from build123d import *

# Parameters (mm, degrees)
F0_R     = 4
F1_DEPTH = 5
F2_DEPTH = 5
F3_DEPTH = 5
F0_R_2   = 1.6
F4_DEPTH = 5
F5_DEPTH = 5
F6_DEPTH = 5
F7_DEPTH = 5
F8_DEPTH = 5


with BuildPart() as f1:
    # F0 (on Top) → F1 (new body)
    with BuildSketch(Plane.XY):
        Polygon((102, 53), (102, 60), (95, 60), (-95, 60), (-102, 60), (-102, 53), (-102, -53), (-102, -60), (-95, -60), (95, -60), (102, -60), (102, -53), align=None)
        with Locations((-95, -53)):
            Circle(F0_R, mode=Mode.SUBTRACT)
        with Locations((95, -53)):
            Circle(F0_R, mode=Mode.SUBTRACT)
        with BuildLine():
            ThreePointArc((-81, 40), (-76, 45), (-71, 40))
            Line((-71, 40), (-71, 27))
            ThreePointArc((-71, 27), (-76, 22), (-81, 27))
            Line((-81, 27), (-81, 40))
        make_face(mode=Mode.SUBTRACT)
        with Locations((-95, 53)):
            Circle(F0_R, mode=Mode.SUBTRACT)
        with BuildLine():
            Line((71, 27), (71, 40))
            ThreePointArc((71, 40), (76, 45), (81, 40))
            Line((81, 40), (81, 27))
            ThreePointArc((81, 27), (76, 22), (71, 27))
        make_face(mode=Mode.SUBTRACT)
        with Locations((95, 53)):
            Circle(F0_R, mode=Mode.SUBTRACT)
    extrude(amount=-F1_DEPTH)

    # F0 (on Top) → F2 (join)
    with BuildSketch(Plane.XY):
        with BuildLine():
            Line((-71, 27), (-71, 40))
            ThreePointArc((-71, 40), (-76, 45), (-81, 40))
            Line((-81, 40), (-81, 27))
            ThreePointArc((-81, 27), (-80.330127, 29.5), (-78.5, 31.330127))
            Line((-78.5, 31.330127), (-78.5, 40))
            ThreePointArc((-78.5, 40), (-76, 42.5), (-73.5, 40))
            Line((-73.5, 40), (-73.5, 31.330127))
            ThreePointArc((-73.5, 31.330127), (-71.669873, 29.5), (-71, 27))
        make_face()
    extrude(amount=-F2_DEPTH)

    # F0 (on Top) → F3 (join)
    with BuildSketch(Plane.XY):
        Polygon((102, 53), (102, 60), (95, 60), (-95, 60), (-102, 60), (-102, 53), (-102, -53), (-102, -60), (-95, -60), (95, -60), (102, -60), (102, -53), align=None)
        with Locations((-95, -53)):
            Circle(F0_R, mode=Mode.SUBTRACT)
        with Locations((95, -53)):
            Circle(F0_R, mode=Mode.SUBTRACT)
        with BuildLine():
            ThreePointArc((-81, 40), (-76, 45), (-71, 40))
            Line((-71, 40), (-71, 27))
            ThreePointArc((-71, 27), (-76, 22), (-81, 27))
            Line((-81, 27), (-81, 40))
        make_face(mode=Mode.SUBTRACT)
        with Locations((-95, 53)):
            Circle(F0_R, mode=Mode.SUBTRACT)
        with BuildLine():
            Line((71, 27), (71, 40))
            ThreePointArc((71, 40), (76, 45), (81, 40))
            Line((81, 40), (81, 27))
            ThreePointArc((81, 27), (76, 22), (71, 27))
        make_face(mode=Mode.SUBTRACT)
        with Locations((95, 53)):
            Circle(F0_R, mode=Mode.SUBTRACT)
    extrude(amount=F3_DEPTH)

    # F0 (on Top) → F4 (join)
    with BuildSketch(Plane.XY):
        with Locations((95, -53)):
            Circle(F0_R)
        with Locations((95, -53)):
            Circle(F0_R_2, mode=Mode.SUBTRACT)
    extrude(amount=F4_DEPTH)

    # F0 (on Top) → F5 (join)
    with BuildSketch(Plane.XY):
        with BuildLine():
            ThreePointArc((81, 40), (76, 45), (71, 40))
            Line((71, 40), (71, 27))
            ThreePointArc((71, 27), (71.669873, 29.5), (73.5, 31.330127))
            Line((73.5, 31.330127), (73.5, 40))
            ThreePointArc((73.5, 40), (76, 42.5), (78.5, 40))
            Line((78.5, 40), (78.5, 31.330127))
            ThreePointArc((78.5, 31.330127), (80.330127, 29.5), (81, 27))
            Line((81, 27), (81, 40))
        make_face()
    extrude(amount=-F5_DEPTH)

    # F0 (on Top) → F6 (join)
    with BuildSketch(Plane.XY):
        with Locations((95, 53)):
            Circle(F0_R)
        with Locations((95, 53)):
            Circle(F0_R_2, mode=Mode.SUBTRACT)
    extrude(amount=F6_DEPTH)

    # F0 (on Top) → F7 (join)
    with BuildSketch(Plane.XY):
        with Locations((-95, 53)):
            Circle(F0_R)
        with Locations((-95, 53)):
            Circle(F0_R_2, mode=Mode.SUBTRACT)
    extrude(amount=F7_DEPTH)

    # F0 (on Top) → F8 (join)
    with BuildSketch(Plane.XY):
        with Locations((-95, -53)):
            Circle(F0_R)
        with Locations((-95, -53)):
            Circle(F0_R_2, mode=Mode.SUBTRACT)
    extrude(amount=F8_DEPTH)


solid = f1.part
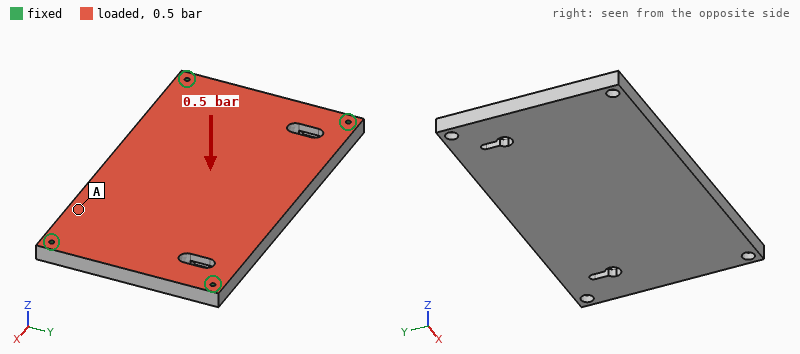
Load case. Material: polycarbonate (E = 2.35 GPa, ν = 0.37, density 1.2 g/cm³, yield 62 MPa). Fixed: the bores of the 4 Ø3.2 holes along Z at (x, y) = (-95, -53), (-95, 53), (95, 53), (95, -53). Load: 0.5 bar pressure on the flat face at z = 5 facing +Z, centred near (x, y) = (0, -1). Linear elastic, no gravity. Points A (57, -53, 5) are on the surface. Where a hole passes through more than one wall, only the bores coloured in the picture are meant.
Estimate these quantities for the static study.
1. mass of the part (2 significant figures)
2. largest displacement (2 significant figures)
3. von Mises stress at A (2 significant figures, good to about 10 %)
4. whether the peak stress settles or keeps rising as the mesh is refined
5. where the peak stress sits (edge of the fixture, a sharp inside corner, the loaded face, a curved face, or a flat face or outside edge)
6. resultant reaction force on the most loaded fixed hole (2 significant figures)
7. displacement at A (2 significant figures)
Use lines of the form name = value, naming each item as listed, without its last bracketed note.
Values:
mass of the part = 290 g
largest displacement = 2.4 mm
von Mises stress at A = 3.6 MPa
whether the peak stress settles or keeps rising as the mesh is refined = keeps rising
where the peak stress sits = edge of the fixture
resultant reaction force on the most loaded fixed hole = 610 N
displacement at A = 1.3 mm
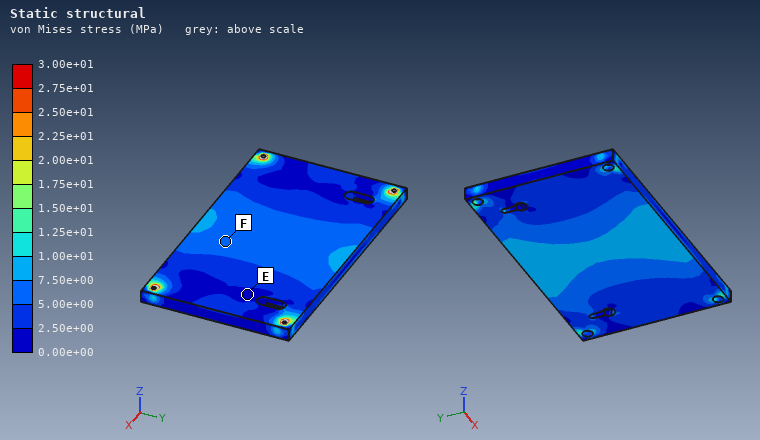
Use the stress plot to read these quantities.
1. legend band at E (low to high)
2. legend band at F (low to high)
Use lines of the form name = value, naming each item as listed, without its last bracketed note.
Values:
legend band at E = 0.00e+00 to 2.50e+00 MPa
legend band at F = 5.00e+00 to 7.50e+00 MPa
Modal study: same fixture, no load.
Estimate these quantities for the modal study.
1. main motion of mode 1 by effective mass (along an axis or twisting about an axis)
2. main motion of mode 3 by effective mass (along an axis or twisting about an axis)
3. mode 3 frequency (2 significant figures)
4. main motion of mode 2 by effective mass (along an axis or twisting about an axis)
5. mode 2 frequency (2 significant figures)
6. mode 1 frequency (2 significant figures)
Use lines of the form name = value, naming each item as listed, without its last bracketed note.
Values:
main motion of mode 1 by effective mass = along Z
main motion of mode 3 by effective mass = twisting about Y
mode 3 frequency = 670 Hz
main motion of mode 2 by effective mass = twisting about X
mode 2 frequency = 460 Hz
mode 1 frequency = 240 Hz
